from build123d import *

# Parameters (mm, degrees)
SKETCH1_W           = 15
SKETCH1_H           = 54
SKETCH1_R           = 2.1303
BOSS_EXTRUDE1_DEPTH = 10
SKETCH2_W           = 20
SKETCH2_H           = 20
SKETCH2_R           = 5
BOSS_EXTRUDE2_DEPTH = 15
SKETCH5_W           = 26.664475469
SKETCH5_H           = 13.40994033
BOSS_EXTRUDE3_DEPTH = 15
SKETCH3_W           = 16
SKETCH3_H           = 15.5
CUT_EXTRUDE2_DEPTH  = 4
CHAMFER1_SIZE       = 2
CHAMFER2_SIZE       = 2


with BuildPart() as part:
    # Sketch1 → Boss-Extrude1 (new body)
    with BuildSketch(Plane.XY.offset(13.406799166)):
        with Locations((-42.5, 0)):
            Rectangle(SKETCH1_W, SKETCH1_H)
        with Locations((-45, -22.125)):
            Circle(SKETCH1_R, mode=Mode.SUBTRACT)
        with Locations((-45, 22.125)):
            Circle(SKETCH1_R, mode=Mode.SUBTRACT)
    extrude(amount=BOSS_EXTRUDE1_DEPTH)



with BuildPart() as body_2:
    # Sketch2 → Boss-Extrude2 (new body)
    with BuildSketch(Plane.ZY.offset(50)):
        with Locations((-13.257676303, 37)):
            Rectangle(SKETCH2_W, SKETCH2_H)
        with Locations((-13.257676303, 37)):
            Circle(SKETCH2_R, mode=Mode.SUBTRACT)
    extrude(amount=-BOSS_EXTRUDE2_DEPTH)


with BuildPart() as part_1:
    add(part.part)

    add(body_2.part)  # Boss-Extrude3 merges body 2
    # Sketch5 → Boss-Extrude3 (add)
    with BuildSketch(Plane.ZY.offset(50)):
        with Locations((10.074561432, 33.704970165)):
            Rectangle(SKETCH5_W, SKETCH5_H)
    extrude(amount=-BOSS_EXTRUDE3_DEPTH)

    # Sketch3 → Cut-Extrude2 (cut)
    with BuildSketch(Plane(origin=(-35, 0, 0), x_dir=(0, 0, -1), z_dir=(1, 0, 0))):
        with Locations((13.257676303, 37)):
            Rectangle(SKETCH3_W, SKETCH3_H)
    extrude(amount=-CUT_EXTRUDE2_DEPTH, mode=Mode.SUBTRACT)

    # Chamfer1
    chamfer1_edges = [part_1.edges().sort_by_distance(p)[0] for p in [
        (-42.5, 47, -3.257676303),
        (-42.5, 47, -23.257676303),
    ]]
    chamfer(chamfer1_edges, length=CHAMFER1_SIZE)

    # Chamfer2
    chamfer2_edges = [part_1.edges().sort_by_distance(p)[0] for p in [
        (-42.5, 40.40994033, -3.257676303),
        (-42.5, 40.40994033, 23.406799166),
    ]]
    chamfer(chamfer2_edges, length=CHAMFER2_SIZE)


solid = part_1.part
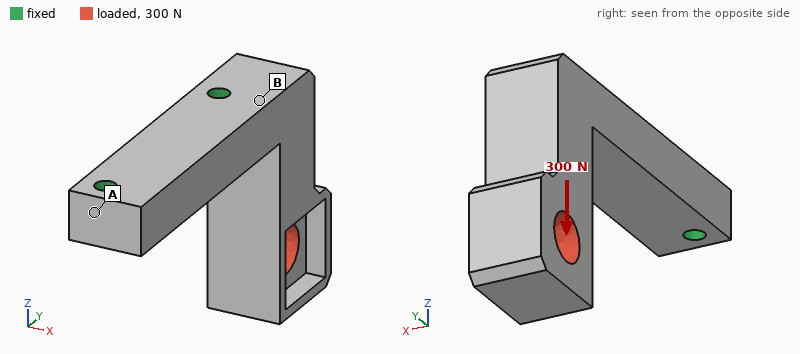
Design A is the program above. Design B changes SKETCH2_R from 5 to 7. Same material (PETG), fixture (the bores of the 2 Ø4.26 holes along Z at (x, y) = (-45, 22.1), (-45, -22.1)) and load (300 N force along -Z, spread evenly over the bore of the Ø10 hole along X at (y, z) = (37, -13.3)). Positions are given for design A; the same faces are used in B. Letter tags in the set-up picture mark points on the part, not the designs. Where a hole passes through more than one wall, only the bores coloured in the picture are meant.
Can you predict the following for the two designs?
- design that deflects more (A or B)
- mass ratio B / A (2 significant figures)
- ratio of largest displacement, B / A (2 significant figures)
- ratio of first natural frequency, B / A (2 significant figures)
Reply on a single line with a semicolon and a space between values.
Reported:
B; 0.95; 1.1; 1.1
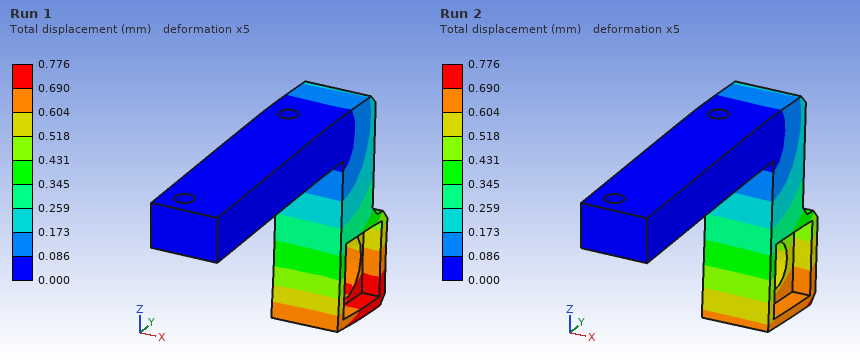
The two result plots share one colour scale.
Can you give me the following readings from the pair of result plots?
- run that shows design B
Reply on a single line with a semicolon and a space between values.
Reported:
Run 1
